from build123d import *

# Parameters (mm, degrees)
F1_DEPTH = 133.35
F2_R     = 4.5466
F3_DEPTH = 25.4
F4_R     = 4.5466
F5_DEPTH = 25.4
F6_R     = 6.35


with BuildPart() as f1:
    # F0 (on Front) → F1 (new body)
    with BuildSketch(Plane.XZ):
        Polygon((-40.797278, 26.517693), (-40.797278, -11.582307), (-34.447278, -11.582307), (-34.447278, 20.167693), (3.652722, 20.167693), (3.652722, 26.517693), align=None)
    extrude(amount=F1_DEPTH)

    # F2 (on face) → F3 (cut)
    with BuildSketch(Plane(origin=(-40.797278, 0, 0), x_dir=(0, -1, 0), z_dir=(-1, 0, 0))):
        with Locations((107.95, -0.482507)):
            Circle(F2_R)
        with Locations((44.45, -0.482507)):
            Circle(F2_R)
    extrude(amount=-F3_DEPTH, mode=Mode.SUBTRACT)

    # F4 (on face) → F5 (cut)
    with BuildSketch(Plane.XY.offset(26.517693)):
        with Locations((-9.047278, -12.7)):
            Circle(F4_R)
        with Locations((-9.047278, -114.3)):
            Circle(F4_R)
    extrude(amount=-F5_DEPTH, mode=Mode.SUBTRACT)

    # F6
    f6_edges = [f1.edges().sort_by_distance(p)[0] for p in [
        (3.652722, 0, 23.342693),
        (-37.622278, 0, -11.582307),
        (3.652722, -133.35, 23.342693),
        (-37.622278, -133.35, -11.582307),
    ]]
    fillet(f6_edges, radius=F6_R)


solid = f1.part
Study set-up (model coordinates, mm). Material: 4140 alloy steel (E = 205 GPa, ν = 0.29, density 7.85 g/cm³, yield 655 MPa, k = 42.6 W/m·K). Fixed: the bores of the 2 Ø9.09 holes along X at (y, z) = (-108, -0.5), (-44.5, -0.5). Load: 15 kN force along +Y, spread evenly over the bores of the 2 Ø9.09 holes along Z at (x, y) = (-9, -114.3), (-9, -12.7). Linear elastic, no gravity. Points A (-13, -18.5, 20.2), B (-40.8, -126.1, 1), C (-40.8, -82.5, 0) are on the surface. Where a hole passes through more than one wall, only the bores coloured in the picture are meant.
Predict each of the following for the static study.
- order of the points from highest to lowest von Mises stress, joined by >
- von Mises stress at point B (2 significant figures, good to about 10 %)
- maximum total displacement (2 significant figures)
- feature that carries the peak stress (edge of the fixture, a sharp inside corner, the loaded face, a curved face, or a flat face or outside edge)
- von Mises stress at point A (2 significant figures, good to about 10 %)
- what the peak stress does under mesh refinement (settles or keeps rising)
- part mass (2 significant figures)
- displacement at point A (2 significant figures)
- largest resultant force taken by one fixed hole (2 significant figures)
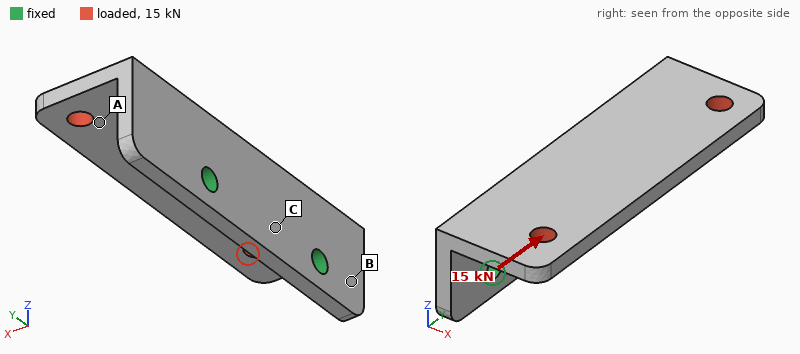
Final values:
B > A > C
130 MPa
0.28 mm
edge of the fixture
74 MPa
keeps rising
490 g
0.18 mm
11 kN
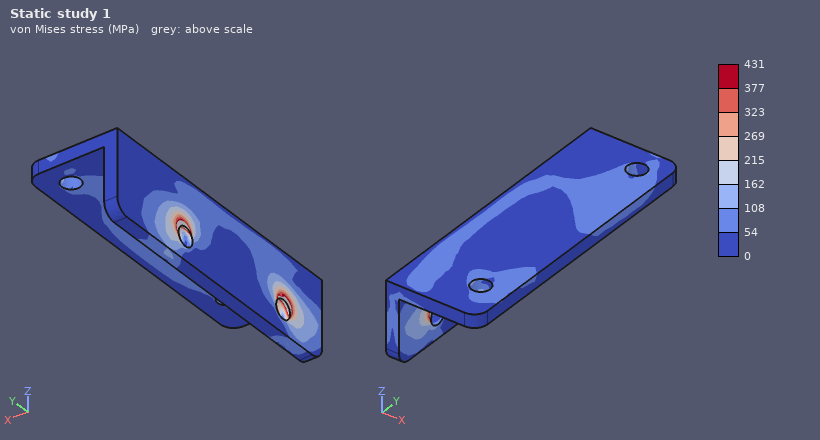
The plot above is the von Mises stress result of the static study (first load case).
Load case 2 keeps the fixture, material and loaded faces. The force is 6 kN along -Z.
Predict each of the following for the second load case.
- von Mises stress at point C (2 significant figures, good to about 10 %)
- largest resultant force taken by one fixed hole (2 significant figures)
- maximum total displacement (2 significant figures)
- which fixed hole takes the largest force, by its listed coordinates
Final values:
72 MPa
4.1 kN
0.58 mm
(-44.5, -0.5)
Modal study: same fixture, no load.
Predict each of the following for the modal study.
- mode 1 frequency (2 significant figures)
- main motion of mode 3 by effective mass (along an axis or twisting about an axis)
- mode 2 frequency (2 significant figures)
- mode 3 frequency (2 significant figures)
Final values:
1500 Hz
along X
2200 Hz
3400 Hz
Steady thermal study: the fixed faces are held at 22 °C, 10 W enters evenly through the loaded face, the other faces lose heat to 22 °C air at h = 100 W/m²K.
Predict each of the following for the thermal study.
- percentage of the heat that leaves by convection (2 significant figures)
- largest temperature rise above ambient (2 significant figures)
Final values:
75 %
13 K
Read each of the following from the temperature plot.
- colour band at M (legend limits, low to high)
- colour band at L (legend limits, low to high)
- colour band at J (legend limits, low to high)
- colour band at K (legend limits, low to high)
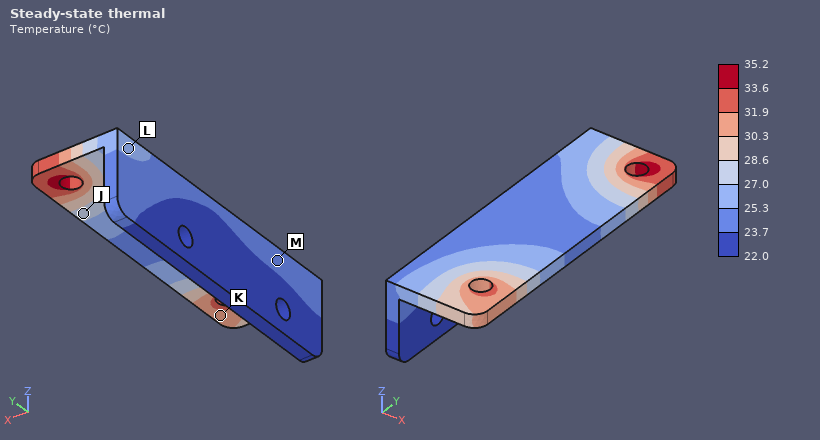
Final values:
23.7 to 25.3 °C
25.3 to 27.0 °C
27.0 to 28.6 °C
30.3 to 31.9 °C
